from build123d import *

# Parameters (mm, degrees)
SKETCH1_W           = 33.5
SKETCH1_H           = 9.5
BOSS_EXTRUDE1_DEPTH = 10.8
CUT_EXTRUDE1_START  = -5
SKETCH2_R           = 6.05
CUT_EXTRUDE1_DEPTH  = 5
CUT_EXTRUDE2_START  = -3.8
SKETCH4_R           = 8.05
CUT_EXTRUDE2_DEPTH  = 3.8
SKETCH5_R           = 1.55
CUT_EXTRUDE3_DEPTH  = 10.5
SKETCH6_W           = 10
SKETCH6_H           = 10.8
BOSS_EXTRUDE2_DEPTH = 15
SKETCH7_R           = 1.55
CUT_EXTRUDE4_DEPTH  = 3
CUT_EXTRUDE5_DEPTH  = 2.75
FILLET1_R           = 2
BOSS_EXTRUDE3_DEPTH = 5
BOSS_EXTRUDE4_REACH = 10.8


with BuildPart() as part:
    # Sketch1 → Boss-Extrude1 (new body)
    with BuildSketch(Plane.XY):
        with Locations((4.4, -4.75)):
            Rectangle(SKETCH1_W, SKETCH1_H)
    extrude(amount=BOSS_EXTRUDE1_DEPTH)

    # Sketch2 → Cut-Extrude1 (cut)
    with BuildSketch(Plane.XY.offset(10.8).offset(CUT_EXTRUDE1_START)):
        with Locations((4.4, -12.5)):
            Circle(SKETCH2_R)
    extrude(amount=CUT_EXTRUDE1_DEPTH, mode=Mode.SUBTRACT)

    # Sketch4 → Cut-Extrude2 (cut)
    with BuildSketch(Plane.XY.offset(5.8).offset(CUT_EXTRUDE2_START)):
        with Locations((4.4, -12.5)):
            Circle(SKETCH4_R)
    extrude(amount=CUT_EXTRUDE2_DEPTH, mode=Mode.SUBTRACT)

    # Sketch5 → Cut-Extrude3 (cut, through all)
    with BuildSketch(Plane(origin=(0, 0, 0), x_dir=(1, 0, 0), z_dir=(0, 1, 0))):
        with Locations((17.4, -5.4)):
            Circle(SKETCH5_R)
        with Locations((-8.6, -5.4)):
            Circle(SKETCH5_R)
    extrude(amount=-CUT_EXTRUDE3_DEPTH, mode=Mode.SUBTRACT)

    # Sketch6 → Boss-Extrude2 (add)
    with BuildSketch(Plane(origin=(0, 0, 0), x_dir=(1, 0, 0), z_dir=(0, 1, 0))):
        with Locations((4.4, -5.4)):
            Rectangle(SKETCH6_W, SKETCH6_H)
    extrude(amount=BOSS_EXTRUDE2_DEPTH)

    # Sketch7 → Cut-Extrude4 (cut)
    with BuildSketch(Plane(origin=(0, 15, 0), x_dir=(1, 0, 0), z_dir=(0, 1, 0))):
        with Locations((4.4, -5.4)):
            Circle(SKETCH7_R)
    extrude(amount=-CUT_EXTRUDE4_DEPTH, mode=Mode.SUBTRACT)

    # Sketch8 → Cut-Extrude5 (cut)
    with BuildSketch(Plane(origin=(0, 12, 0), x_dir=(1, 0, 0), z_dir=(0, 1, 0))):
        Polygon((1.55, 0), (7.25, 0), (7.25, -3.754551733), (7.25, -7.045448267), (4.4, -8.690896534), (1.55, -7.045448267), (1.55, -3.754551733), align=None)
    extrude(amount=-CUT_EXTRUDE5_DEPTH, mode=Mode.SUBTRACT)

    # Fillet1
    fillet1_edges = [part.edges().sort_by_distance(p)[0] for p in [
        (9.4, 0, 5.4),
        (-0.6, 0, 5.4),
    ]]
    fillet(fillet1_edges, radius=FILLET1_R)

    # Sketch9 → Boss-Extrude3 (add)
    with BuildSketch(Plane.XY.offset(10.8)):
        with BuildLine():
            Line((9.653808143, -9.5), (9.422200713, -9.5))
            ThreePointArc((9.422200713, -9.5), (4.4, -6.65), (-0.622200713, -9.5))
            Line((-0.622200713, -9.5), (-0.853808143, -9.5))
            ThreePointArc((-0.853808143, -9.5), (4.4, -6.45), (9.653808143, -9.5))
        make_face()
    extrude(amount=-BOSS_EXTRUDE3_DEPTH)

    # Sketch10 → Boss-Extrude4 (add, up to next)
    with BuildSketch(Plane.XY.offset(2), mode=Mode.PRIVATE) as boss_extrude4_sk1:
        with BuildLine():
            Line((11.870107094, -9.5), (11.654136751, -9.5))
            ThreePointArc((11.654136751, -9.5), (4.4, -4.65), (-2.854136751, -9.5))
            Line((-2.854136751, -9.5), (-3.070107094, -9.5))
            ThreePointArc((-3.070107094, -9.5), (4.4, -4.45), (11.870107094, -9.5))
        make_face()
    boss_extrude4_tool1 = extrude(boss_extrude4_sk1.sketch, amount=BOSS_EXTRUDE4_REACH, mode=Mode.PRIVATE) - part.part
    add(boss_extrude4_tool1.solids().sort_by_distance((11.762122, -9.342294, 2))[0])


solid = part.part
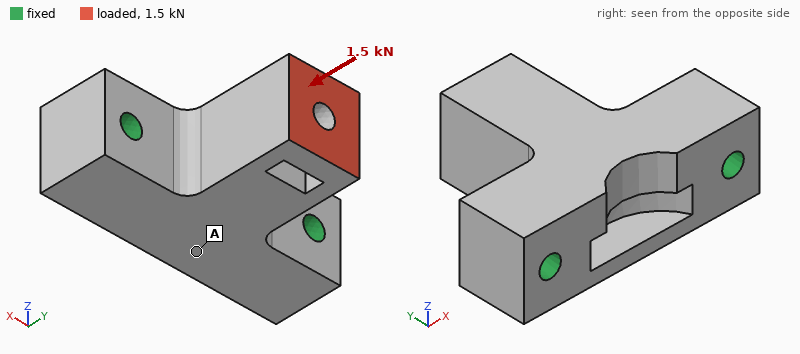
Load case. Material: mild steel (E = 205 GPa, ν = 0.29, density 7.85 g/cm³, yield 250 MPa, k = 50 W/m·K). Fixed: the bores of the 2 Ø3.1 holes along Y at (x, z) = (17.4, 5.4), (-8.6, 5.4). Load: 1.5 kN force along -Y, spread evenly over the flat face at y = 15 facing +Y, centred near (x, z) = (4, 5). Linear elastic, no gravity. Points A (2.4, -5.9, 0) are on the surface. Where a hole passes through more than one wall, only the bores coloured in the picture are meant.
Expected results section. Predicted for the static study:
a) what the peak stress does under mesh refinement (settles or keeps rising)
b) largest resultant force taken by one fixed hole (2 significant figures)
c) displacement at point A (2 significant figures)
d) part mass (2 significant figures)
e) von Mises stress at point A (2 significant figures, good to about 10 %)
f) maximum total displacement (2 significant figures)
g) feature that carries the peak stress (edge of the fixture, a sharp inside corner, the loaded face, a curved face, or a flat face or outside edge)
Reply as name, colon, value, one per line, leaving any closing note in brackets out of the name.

what the peak stress does under mesh refinement: keeps rising
largest resultant force taken by one fixed hole: 820 N
displacement at point A: 1.6 µm
part mass: 35 g
von Mises stress at point A: 7.8 MPa
maximum total displacement: 4.4 µm
feature that carries the peak stress: edge of the fixture
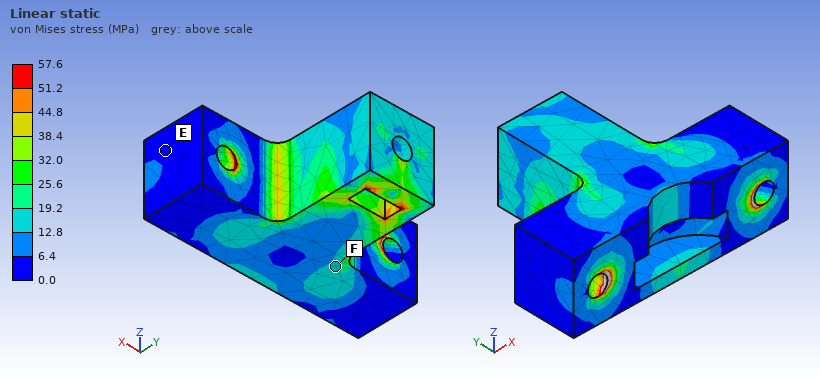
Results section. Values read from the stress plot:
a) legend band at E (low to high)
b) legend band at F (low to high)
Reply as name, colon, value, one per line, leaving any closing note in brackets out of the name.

legend band at E: 0.0 to 6.4 MPa
legend band at F: 12.8 to 19.2 MPa
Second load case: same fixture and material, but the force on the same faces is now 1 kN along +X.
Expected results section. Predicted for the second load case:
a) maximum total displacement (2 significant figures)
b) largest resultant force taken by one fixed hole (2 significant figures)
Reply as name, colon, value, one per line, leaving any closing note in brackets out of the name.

maximum total displacement: 17 µm
largest resultant force taken by one fixed hole: 1.1 kN
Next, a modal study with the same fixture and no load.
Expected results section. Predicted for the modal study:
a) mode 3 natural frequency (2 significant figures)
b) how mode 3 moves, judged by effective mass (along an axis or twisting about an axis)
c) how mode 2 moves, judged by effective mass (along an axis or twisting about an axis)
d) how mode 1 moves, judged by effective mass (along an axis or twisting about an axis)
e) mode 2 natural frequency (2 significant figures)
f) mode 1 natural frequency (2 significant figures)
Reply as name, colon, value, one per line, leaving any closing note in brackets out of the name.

mode 3 natural frequency: 33 kHz
how mode 3 moves, judged by effective mass: along Y
how mode 2 moves, judged by effective mass: along X
how mode 1 moves, judged by effective mass: along Z
mode 2 natural frequency: 22 kHz
mode 1 natural frequency: 13 kHz
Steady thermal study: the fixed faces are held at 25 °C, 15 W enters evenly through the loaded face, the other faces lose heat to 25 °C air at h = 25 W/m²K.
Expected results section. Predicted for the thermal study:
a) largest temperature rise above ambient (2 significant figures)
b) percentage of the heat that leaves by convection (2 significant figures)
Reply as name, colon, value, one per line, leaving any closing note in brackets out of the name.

largest temperature rise above ambient: 74 K
percentage of the heat that leaves by convection: 7.0 %
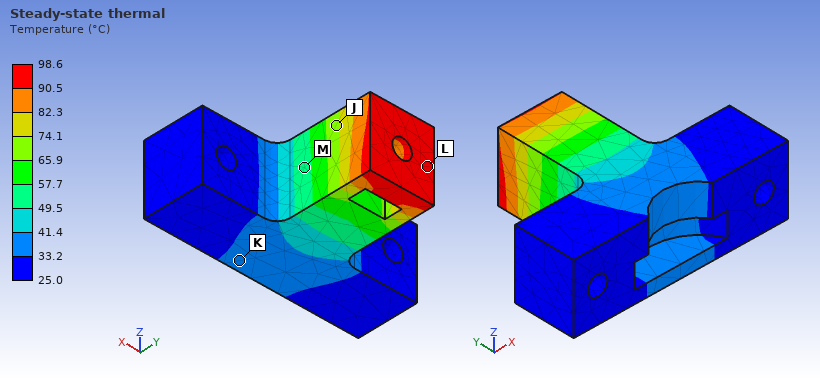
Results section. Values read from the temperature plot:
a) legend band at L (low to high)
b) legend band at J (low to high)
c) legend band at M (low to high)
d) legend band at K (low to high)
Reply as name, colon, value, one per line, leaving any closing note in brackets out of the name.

legend band at L: 90.5 to 98.6 °C
legend band at J: 65.9 to 74.1 °C
legend band at M: 49.5 to 57.7 °C
legend band at K: 33.2 to 41.4 °C
